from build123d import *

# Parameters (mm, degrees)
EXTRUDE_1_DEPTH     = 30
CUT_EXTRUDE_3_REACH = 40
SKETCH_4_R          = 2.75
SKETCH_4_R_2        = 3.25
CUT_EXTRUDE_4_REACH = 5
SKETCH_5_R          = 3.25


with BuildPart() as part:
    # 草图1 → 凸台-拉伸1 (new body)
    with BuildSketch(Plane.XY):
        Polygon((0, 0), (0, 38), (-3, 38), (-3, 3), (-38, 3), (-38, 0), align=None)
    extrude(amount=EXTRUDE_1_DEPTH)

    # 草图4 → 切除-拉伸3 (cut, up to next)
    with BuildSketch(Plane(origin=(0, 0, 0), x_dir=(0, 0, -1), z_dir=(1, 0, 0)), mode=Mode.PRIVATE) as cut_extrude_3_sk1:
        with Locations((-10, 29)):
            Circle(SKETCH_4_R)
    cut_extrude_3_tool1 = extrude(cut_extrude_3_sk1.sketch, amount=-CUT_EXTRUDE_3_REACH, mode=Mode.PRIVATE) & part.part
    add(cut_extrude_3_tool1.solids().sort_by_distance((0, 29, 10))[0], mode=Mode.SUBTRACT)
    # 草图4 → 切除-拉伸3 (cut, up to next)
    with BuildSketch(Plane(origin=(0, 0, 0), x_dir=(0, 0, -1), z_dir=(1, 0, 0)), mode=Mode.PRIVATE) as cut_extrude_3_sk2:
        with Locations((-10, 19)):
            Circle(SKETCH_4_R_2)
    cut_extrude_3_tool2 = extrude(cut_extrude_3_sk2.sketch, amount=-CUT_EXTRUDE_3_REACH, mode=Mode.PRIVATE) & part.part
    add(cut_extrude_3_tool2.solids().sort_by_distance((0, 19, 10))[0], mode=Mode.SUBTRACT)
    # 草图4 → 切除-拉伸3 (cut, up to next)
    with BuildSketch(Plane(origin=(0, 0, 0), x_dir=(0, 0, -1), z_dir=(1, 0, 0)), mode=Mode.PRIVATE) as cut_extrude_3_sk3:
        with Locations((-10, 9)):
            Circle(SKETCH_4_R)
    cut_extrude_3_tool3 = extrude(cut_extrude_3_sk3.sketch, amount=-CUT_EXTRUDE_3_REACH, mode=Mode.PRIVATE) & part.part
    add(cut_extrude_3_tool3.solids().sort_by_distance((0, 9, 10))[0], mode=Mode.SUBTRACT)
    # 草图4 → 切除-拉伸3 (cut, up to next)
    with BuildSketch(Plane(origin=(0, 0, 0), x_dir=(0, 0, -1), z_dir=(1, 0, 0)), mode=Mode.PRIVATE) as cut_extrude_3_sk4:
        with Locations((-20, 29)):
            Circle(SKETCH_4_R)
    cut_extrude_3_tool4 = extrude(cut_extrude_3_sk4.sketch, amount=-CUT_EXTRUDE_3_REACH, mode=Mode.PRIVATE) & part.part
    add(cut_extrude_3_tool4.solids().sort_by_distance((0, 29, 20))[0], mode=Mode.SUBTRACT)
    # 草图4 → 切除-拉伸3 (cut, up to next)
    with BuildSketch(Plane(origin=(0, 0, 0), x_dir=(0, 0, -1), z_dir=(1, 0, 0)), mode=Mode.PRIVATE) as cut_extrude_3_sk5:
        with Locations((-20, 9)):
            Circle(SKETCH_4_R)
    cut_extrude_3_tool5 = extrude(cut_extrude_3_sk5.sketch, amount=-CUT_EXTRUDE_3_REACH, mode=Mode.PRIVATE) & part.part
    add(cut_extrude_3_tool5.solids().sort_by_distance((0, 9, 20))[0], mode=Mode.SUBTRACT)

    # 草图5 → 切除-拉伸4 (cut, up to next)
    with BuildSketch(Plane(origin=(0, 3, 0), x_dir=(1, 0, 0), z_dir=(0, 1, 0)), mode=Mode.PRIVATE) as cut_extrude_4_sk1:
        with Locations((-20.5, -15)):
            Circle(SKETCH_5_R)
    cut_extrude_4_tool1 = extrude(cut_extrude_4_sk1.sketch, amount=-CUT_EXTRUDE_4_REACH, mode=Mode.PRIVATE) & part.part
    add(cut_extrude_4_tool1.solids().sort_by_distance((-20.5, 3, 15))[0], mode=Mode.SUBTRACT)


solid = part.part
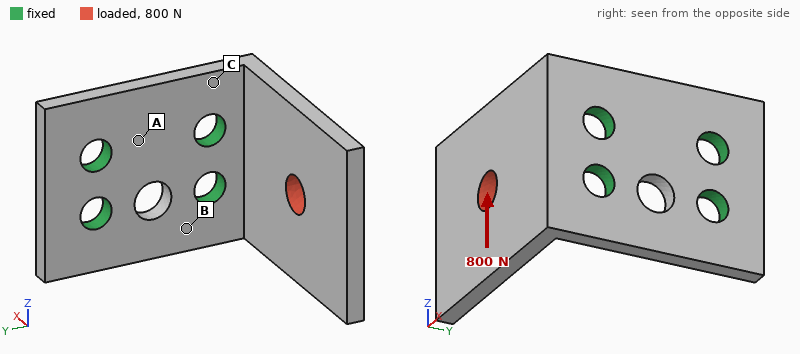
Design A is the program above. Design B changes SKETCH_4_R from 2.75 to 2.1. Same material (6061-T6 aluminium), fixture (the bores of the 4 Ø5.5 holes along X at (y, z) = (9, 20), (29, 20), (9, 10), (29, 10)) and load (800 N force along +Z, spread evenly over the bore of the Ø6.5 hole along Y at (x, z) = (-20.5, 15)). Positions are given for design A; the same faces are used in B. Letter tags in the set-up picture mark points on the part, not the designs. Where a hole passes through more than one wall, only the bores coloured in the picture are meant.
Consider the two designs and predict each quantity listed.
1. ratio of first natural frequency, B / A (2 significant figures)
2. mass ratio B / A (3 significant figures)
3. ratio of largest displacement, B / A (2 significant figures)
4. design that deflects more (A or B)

0.97
1.02
1.2
B
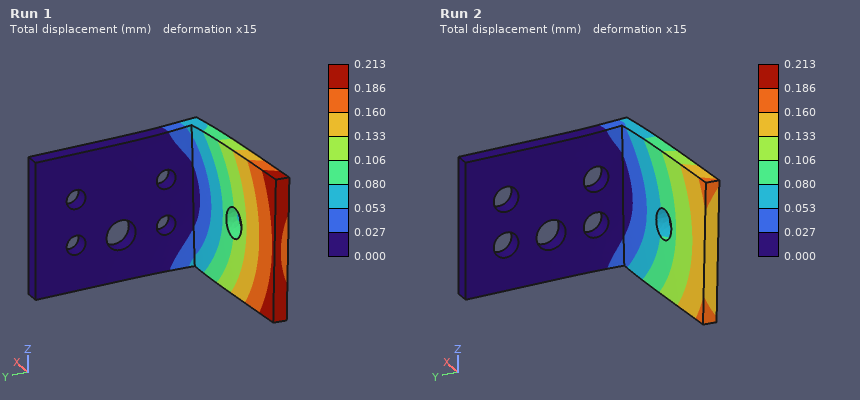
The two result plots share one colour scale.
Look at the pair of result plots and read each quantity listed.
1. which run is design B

Run 1
